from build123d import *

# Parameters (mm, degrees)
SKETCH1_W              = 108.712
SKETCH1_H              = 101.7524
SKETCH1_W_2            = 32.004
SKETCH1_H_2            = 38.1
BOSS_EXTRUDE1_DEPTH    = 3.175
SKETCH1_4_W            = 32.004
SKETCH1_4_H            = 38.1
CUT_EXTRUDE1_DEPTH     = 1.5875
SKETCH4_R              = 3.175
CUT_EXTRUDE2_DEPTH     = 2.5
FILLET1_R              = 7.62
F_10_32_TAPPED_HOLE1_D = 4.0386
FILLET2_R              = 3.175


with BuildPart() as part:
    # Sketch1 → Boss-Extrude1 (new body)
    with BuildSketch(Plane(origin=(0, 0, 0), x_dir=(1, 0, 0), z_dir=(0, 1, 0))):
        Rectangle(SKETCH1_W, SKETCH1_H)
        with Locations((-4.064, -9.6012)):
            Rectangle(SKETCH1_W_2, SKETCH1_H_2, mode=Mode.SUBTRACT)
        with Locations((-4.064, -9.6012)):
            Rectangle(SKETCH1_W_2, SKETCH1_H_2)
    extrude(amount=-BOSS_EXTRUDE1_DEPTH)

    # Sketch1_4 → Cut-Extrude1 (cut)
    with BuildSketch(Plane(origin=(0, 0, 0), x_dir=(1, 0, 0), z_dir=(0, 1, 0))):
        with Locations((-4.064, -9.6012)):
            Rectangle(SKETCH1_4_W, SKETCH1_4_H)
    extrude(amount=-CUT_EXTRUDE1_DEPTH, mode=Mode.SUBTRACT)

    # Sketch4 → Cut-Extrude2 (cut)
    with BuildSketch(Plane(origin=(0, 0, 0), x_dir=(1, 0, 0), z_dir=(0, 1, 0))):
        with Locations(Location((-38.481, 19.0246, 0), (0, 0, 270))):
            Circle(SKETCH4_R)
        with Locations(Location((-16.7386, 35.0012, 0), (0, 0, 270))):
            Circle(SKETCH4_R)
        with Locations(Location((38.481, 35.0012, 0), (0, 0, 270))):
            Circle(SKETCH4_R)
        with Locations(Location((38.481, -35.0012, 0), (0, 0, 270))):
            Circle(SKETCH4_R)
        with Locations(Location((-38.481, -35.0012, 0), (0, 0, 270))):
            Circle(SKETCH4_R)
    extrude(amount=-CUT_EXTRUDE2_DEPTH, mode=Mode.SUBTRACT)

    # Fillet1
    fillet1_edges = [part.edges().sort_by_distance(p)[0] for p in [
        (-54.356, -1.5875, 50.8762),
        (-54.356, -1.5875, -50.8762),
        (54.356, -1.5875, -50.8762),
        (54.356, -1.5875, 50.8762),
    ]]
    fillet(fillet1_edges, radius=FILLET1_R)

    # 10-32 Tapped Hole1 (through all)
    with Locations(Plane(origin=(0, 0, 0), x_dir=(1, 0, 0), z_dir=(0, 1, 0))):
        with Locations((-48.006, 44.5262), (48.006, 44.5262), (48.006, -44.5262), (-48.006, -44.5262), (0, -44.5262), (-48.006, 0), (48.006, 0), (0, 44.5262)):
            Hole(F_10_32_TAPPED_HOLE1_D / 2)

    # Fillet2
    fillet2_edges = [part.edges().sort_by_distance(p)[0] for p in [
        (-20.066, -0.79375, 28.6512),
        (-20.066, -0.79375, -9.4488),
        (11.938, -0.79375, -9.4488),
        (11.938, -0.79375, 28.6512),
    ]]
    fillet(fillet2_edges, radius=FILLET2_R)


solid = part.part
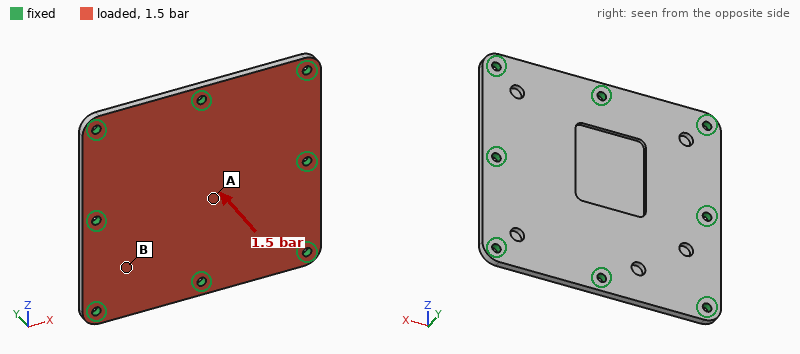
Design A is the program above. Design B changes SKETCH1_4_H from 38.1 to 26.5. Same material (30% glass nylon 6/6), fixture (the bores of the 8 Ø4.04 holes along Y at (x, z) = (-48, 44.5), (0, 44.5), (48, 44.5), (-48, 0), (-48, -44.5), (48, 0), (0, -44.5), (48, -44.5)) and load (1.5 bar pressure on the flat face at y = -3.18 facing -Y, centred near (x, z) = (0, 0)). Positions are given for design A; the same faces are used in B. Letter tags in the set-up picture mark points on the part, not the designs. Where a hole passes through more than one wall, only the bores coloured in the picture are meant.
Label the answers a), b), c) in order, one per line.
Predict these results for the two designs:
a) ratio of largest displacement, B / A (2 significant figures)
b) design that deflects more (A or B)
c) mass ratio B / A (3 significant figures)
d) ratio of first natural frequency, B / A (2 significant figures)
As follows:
a) 0.92
b) A
c) 1.02
d) 1.00
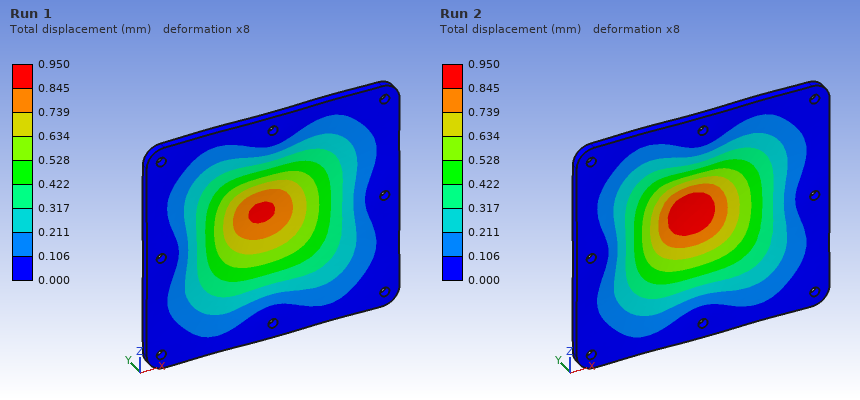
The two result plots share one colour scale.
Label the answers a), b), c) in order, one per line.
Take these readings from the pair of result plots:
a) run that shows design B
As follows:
a) Run 1
